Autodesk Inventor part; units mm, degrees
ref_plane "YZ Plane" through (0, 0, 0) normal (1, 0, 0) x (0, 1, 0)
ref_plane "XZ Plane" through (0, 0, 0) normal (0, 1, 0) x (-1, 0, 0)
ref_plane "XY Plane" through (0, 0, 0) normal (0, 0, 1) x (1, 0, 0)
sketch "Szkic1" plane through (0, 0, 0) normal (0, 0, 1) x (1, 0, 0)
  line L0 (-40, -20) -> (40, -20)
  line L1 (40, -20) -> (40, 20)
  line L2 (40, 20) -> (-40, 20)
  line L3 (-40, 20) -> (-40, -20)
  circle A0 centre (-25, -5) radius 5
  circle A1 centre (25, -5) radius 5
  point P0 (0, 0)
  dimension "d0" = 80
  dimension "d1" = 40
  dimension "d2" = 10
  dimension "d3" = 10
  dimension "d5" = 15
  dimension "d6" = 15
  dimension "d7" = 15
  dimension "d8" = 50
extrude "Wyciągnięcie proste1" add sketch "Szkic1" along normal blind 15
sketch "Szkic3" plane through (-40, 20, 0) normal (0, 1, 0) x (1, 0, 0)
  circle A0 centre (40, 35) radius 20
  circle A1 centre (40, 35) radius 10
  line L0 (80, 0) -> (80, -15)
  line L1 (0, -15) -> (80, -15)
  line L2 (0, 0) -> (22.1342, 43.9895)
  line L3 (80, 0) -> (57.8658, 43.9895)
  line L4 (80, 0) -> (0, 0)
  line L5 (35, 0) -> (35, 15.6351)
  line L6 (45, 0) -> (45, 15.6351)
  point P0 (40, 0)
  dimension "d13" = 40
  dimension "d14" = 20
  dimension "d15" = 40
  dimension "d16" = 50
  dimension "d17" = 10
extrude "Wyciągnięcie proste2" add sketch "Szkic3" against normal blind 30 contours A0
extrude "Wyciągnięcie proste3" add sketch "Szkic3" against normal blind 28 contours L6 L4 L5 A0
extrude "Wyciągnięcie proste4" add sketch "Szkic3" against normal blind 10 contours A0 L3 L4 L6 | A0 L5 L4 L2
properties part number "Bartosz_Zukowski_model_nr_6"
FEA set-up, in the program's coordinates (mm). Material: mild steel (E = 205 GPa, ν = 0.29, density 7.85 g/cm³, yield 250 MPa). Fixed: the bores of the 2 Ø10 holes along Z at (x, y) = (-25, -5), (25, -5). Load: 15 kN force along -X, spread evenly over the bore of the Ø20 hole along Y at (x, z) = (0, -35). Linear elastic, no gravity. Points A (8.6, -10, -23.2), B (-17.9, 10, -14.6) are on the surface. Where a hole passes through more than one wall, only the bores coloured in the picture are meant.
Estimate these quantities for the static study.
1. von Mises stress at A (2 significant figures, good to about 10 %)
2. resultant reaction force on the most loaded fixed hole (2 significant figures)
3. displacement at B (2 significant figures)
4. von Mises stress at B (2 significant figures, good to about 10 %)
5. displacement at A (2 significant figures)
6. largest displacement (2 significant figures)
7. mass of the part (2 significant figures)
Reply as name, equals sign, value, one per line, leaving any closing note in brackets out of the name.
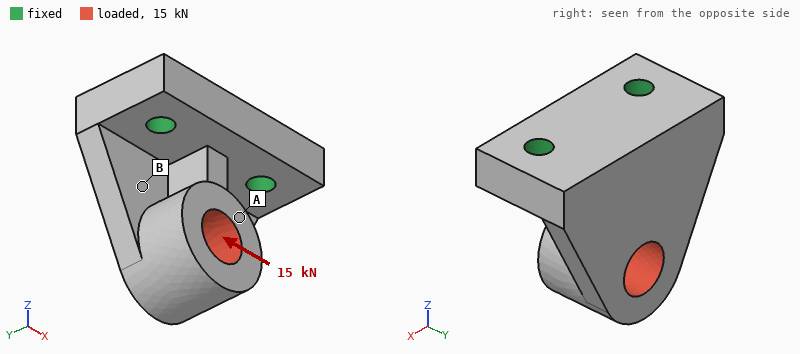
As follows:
von Mises stress at A = 24 MPa
resultant reaction force on the most loaded fixed hole = 14 kN
displacement at B = 25 µm
von Mises stress at B = 73 MPa
displacement at A = 49 µm
largest displacement = 78 µm
mass of the part = 730 g
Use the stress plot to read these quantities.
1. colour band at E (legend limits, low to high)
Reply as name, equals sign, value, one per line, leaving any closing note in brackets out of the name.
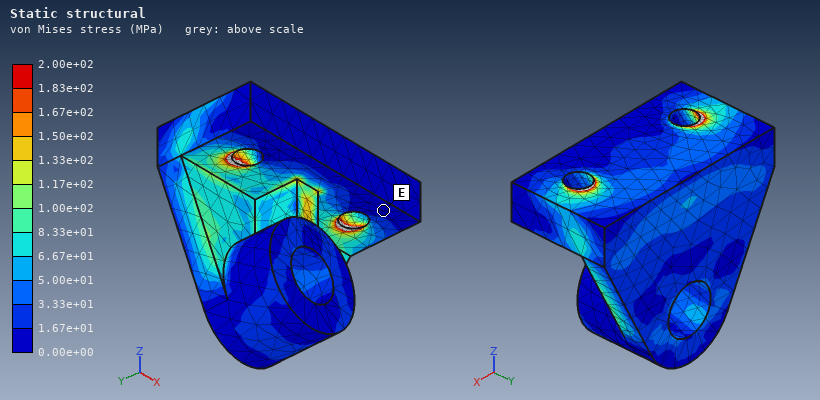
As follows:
colour band at E = 0.00e+00 to 1.67e+01 MPa
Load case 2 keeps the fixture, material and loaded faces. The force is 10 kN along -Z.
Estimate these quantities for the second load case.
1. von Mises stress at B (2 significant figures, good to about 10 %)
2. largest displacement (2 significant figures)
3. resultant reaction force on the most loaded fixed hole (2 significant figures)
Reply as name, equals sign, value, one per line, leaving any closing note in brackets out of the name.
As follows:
von Mises stress at B = 23 MPa
largest displacement = 15 µm
resultant reaction force on the most loaded fixed hole = 5.0 kN
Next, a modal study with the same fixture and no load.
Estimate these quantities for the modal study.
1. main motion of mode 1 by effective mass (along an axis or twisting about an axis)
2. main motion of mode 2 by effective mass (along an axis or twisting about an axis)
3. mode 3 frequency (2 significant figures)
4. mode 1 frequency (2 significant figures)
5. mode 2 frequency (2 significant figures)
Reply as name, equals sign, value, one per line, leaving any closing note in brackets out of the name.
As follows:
main motion of mode 1 by effective mass = along Y
main motion of mode 2 by effective mass = along X
mode 3 frequency = 8800 Hz
mode 1 frequency = 3100 Hz
mode 2 frequency = 5100 Hz
